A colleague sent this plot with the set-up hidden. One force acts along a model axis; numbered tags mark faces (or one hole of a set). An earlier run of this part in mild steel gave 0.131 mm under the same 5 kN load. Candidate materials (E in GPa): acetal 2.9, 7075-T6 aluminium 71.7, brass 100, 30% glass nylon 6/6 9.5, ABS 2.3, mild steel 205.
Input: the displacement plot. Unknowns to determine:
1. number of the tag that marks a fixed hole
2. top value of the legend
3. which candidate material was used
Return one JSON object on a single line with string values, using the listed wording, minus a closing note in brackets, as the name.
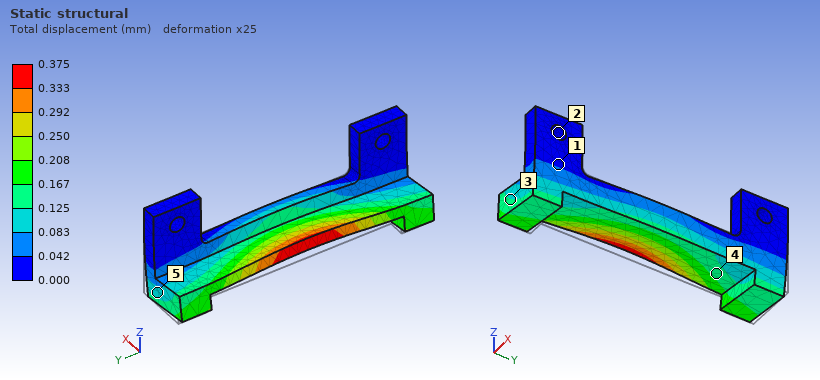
{"number of the tag that marks a fixed hole": "2", "top value of the legend": "0.375 mm", "which candidate material was used": "7075-T6 aluminium"}
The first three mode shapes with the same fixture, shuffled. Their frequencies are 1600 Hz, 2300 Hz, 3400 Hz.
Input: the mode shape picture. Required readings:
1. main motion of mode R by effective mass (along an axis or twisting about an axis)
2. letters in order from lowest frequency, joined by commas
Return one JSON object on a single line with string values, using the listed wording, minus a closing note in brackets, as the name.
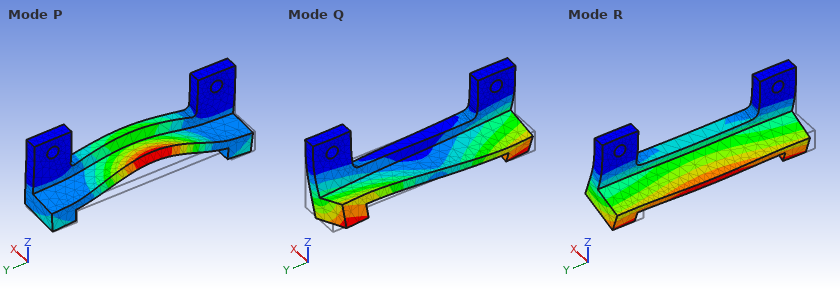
{"main motion of mode R by effective mass": "along X", "letters in order from lowest frequency, joined by commas": "R, Q, P"}
